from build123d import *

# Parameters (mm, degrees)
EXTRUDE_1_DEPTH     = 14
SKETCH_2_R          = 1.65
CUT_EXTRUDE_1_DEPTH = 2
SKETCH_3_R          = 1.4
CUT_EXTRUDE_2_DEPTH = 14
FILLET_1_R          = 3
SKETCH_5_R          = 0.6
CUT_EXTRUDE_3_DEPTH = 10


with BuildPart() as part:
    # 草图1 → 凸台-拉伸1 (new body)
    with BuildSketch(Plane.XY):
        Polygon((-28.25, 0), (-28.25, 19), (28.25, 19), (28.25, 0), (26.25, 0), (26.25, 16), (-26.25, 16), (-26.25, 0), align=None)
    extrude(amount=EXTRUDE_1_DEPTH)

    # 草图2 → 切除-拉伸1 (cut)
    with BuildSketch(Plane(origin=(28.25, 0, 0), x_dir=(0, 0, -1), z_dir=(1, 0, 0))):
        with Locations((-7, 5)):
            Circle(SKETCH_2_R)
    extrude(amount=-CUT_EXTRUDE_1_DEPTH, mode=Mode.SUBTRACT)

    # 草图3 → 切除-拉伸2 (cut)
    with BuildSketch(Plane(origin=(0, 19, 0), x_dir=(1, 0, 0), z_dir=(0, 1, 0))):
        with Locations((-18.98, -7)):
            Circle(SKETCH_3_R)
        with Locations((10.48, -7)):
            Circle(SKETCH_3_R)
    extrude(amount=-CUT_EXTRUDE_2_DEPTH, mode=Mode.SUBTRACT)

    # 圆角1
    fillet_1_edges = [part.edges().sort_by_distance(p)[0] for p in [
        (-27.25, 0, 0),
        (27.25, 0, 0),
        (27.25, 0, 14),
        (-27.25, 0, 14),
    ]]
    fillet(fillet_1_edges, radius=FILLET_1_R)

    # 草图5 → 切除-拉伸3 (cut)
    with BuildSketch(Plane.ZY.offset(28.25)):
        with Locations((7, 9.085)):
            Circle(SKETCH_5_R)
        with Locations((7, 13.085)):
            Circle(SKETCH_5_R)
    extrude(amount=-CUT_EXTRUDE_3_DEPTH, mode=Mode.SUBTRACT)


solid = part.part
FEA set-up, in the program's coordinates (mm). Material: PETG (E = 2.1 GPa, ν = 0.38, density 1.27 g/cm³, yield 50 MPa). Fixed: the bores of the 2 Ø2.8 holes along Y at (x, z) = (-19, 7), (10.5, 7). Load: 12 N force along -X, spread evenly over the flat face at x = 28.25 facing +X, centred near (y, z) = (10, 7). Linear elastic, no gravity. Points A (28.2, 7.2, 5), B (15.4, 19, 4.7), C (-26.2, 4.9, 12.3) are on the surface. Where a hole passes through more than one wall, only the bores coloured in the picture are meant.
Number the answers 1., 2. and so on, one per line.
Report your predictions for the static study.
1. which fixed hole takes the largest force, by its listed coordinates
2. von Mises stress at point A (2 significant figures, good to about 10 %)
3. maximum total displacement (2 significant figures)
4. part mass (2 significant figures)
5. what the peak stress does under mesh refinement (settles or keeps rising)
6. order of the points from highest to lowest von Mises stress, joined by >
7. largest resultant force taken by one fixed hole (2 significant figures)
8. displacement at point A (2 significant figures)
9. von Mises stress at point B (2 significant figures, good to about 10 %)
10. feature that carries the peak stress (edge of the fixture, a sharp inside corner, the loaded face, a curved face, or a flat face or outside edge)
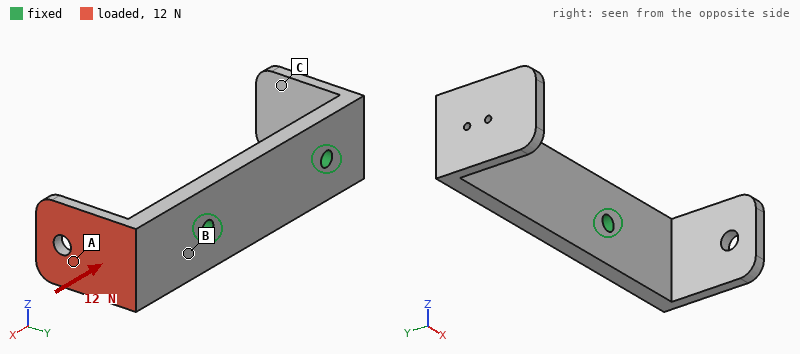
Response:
1. (10.5, 7)
2. 1.8 MPa
3. 0.72 mm
4. 4.1 g
5. keeps rising
6. B > A > C
7. 11 N
8. 0.43 mm
9. 3.9 MPa
10. edge of the fixture
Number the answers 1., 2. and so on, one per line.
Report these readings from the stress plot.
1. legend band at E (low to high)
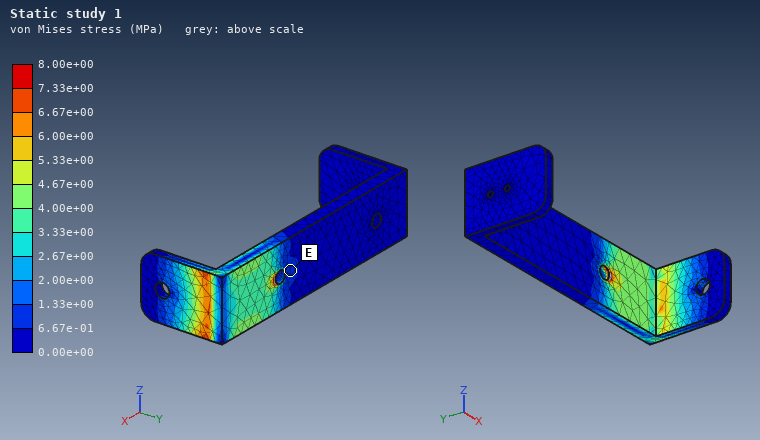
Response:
1. 6.67e-01 to 1.33e+00 MPa
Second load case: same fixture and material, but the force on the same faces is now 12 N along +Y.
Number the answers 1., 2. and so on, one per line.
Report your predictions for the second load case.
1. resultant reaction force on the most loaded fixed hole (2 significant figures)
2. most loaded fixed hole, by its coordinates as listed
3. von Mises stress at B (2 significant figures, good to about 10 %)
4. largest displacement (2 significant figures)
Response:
1. 13 N
2. (10.5, 7)
3. 6.9 MPa
4. 0.63 mm
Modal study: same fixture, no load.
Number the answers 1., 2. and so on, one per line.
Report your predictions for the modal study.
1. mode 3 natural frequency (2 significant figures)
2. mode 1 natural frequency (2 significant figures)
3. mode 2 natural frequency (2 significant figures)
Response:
1. 1300 Hz
2. 850 Hz
3. 1200 Hz
